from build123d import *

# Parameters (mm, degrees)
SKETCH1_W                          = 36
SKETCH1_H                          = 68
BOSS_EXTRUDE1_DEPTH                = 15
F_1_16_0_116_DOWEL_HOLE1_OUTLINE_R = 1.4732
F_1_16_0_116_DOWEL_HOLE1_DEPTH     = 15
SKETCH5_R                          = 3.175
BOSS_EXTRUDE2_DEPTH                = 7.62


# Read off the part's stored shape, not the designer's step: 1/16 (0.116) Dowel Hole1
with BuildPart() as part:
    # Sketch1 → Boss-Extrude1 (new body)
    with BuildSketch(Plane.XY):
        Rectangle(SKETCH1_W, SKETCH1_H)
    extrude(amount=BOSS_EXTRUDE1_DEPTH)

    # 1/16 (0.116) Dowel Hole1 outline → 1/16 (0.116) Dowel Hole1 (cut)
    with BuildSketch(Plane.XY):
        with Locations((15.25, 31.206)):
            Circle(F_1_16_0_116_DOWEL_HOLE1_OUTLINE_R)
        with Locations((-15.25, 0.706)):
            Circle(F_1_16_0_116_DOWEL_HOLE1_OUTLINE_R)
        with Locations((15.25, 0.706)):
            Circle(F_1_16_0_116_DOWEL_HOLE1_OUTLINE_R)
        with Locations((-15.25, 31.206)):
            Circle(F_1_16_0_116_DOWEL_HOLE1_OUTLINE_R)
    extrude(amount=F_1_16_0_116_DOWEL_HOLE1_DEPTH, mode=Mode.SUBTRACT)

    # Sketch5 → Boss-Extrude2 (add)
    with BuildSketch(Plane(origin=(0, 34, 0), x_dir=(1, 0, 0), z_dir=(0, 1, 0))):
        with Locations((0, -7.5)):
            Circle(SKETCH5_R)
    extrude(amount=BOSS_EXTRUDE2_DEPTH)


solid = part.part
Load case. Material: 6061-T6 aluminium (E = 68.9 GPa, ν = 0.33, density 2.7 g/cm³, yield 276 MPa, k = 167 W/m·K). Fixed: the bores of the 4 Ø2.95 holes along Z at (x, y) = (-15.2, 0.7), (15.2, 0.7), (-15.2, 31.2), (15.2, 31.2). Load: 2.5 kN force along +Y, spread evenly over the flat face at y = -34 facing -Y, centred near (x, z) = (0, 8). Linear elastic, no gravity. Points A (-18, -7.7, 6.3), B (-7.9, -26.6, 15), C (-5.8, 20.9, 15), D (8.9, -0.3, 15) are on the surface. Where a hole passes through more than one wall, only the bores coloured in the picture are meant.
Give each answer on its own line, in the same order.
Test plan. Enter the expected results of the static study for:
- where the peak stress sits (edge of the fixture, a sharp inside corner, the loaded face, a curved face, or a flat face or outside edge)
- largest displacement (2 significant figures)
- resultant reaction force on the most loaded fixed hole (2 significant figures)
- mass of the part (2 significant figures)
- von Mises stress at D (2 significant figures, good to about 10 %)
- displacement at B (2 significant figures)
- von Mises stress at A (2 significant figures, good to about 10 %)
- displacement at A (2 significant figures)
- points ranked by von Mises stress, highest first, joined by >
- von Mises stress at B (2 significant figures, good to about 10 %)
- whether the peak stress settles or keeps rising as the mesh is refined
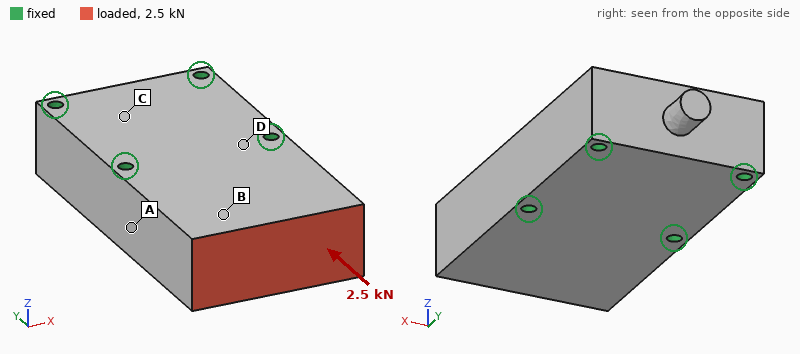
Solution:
edge of the fixture
2.7 µm
1.1 kN
99 g
2.6 MPa
2.2 µm
6.5 MPa
0.83 µm
A > B > D > C
4.6 MPa
keeps rising
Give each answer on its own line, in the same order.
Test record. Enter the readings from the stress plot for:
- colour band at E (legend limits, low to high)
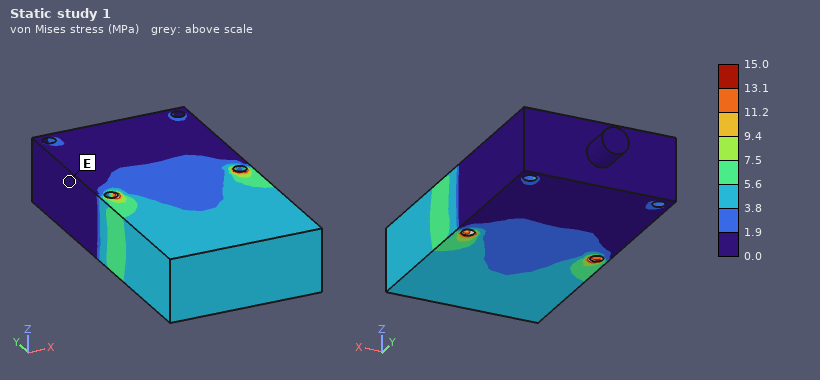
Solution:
0.0 to 1.9 MPa
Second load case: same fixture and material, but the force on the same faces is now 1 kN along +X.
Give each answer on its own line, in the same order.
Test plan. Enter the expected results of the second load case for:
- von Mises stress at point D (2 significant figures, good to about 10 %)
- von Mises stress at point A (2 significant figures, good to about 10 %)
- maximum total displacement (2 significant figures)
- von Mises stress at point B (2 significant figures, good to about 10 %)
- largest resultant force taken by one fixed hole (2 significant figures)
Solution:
2.1 MPa
8.6 MPa
7.4 µm
4.3 MPa
1.2 kN
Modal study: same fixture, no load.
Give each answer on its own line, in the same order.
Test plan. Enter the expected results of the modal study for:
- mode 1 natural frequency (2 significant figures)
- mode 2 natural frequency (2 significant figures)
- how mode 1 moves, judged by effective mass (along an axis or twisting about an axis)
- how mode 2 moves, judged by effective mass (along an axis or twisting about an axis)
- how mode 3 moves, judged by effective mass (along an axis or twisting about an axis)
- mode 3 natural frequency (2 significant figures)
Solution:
7700 Hz
15 kHz
along Z
along X
twisting about Y
16 kHz
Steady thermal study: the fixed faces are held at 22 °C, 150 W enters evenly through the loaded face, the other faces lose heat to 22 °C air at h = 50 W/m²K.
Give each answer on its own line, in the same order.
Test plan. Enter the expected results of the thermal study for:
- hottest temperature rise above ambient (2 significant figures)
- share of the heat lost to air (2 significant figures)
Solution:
62 K
4.2 %
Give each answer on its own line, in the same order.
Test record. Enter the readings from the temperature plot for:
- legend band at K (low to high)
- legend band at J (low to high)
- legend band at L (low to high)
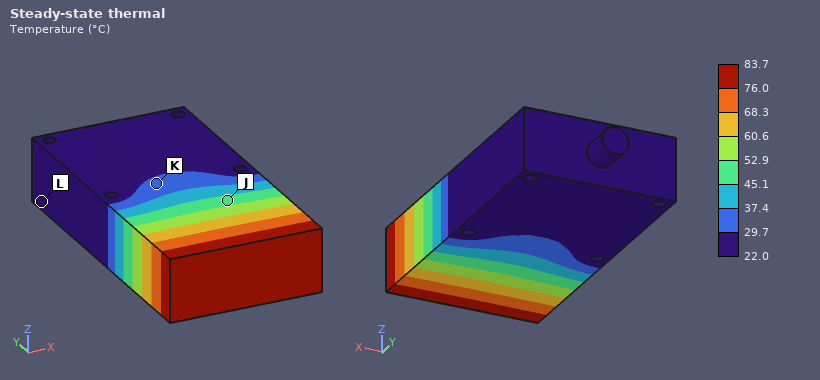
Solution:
29.7 to 37.4 °C
45.1 to 52.9 °C
22.0 to 29.7 °C
